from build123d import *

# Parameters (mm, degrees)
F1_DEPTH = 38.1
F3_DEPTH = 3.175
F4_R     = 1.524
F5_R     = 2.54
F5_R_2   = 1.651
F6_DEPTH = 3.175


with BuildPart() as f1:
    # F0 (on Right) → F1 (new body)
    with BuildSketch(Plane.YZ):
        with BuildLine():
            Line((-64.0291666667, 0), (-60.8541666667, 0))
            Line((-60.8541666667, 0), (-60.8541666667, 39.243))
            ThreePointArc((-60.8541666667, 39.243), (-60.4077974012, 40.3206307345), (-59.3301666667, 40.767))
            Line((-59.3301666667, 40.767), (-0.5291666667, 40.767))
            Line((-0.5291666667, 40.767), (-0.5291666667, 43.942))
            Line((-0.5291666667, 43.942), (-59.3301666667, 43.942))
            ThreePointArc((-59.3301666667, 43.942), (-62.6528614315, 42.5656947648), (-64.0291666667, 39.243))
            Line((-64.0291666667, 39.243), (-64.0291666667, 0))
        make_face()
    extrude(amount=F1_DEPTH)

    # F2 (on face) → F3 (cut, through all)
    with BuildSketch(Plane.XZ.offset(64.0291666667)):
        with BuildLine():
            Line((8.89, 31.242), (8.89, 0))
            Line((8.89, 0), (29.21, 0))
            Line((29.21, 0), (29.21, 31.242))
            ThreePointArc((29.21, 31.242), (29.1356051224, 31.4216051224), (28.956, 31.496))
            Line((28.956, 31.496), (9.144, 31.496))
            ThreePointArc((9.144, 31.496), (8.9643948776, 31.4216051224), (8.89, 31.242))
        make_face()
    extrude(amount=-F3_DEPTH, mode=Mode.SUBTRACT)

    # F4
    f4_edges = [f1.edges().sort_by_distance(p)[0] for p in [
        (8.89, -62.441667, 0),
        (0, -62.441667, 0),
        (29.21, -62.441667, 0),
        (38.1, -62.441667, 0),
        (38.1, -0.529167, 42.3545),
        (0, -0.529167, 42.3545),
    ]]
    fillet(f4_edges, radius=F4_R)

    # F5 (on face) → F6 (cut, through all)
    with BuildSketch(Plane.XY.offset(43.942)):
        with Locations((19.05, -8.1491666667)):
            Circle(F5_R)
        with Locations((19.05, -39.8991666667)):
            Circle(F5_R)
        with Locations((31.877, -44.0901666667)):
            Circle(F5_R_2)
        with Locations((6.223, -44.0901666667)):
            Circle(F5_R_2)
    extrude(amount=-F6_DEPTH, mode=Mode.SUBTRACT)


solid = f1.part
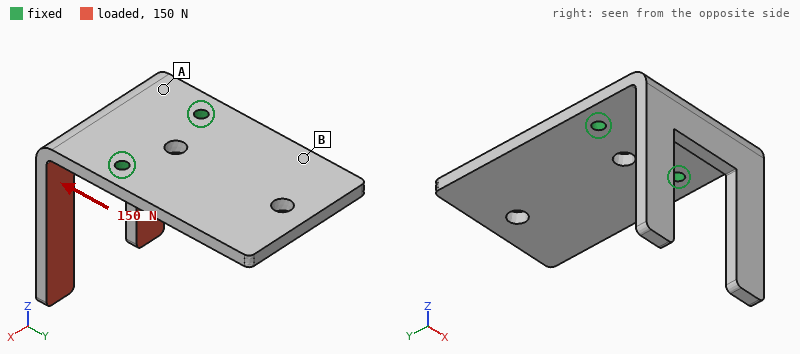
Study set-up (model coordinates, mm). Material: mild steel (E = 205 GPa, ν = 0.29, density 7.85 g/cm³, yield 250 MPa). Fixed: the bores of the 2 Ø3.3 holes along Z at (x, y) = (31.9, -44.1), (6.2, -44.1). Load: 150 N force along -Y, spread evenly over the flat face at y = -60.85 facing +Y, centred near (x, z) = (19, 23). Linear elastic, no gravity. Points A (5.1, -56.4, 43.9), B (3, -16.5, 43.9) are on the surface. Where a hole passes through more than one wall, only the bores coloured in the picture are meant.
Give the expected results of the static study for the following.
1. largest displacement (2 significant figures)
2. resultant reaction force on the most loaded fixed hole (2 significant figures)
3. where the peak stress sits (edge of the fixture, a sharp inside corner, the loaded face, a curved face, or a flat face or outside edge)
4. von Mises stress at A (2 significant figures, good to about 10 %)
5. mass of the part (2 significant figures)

0.20 mm
77 N
a curved face
43 MPa
80 g
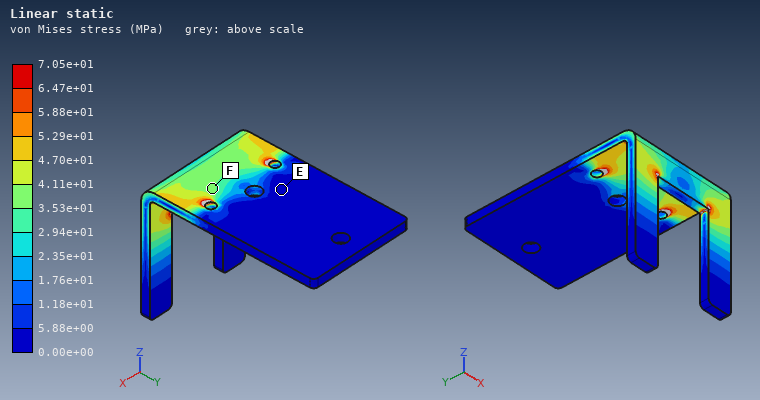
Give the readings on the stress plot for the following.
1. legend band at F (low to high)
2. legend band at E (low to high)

3.53e+01 to 4.11e+01 MPa
0.00e+00 to 5.88e+00 MPa
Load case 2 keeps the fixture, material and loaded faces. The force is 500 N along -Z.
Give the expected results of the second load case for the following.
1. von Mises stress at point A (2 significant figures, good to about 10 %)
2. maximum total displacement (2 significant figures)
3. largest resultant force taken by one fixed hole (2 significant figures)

34 MPa
0.13 mm
250 N
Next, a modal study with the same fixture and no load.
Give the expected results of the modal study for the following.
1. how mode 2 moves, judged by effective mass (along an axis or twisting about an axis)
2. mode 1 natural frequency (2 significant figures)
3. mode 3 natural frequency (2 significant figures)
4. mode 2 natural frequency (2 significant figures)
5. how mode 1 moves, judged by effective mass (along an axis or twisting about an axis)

along Z
1100 Hz
1500 Hz
1400 Hz
along Y
